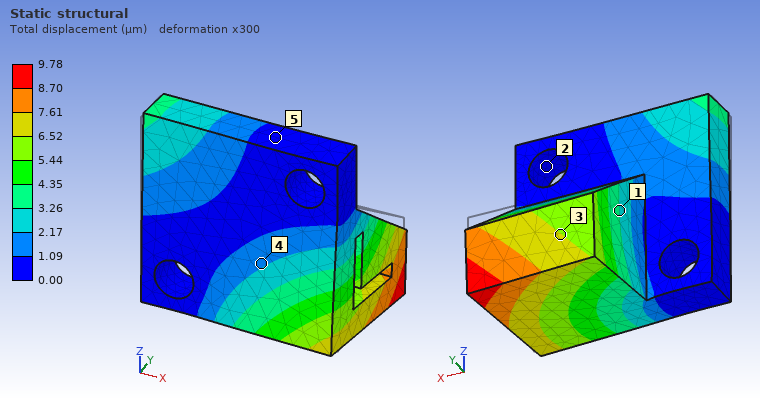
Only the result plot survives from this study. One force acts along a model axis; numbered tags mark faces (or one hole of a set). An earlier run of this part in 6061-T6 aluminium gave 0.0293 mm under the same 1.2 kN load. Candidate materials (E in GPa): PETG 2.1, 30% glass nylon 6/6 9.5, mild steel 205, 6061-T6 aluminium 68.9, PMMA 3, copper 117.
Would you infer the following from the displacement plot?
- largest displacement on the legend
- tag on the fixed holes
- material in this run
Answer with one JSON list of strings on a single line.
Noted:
["9.78 µm", "2", "mild steel"]
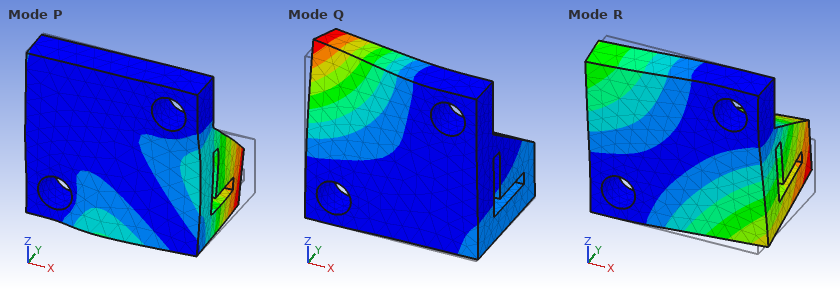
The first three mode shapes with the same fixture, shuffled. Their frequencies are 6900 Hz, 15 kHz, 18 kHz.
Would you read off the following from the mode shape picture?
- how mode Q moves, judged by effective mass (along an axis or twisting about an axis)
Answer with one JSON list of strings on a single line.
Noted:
["along Y"]
